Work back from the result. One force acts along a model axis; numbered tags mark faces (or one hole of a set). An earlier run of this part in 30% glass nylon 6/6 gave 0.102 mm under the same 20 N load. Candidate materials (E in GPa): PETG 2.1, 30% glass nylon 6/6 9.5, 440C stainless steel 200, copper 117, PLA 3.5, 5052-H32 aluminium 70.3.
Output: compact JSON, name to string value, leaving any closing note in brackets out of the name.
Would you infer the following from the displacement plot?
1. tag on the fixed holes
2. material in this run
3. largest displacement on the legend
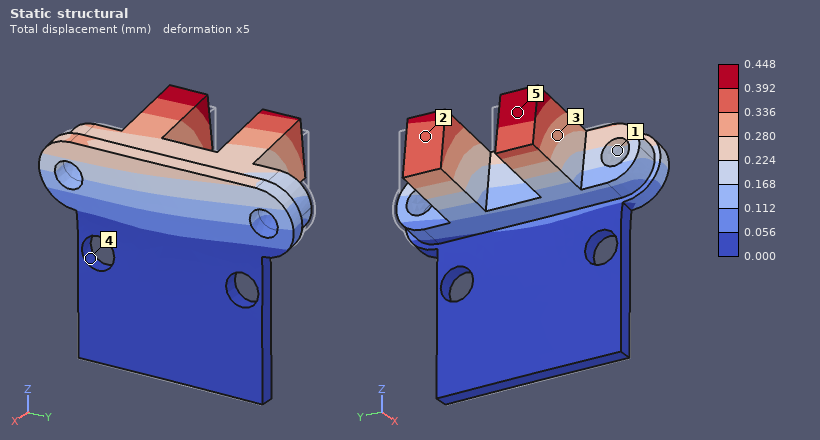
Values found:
{"tag on the fixed holes": "4", "material in this run": "PETG", "largest displacement on the legend": "0.448 mm"}
